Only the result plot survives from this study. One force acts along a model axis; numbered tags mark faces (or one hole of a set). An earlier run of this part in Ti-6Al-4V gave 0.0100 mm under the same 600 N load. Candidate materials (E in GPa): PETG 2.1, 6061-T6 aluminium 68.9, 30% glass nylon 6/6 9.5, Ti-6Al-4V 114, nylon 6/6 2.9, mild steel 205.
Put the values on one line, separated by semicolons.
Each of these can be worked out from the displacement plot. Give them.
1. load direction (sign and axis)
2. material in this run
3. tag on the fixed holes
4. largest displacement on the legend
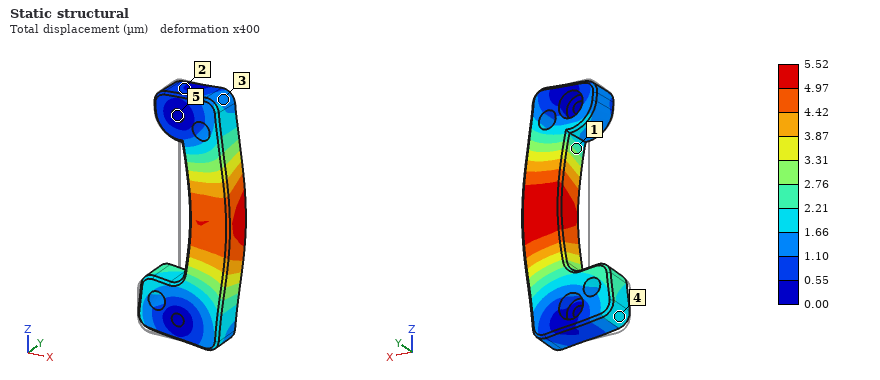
+X; mild steel; 5; 5.52 µm
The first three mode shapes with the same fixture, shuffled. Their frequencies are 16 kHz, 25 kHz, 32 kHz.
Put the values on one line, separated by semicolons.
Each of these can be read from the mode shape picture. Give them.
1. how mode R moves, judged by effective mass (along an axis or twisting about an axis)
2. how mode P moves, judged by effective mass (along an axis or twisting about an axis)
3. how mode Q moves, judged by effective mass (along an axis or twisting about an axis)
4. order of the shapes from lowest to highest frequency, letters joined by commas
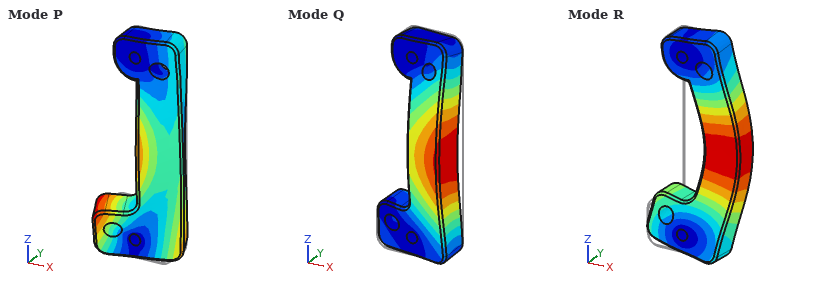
along X; twisting about Z; along Y; Q, R, P
